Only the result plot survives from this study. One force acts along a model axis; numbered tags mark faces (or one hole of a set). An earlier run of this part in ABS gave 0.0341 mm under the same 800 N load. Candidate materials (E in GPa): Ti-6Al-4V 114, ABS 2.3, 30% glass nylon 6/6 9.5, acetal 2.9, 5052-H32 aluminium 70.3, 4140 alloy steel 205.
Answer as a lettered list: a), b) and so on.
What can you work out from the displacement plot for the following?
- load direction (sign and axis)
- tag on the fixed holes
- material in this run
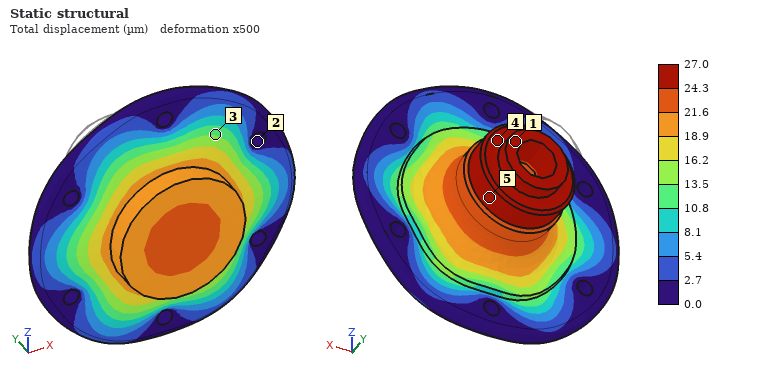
a) -Y
b) 2
c) acetal
